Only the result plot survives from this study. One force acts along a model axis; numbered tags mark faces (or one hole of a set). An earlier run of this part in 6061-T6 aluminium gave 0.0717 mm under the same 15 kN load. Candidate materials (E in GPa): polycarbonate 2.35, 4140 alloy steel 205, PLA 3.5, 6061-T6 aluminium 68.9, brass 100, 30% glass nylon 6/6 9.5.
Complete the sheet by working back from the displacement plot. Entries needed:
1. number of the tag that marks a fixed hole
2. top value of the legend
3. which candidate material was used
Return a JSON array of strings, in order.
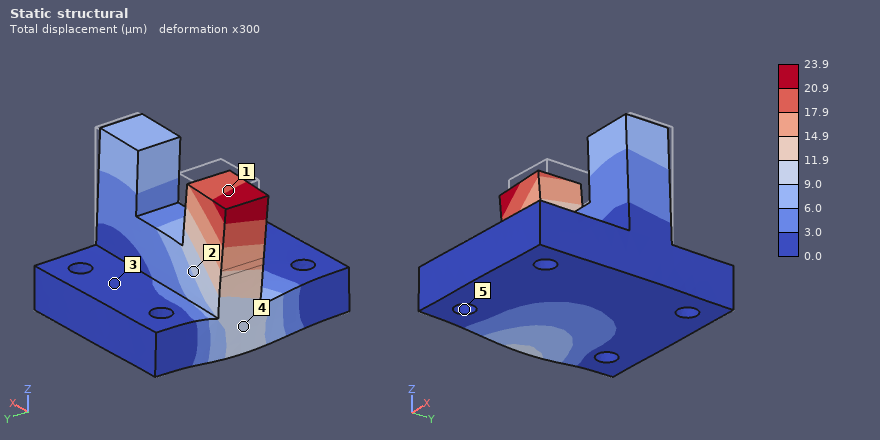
["5", "23.9 µm", "4140 alloy steel"]
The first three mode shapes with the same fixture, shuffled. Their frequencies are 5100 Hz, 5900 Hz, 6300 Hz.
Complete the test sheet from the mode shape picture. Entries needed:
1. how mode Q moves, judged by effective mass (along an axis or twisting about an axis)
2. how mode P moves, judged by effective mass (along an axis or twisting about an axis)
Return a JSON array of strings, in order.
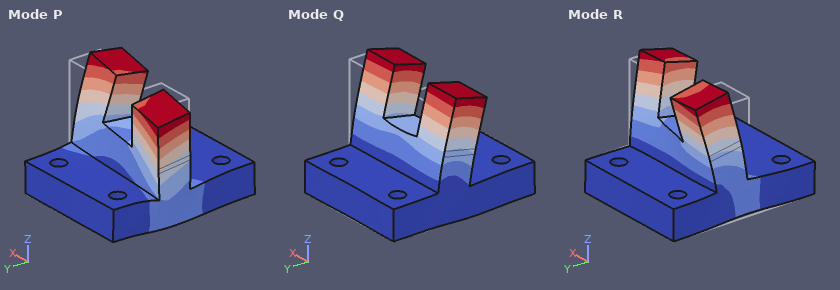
["along Y", "along X"]
